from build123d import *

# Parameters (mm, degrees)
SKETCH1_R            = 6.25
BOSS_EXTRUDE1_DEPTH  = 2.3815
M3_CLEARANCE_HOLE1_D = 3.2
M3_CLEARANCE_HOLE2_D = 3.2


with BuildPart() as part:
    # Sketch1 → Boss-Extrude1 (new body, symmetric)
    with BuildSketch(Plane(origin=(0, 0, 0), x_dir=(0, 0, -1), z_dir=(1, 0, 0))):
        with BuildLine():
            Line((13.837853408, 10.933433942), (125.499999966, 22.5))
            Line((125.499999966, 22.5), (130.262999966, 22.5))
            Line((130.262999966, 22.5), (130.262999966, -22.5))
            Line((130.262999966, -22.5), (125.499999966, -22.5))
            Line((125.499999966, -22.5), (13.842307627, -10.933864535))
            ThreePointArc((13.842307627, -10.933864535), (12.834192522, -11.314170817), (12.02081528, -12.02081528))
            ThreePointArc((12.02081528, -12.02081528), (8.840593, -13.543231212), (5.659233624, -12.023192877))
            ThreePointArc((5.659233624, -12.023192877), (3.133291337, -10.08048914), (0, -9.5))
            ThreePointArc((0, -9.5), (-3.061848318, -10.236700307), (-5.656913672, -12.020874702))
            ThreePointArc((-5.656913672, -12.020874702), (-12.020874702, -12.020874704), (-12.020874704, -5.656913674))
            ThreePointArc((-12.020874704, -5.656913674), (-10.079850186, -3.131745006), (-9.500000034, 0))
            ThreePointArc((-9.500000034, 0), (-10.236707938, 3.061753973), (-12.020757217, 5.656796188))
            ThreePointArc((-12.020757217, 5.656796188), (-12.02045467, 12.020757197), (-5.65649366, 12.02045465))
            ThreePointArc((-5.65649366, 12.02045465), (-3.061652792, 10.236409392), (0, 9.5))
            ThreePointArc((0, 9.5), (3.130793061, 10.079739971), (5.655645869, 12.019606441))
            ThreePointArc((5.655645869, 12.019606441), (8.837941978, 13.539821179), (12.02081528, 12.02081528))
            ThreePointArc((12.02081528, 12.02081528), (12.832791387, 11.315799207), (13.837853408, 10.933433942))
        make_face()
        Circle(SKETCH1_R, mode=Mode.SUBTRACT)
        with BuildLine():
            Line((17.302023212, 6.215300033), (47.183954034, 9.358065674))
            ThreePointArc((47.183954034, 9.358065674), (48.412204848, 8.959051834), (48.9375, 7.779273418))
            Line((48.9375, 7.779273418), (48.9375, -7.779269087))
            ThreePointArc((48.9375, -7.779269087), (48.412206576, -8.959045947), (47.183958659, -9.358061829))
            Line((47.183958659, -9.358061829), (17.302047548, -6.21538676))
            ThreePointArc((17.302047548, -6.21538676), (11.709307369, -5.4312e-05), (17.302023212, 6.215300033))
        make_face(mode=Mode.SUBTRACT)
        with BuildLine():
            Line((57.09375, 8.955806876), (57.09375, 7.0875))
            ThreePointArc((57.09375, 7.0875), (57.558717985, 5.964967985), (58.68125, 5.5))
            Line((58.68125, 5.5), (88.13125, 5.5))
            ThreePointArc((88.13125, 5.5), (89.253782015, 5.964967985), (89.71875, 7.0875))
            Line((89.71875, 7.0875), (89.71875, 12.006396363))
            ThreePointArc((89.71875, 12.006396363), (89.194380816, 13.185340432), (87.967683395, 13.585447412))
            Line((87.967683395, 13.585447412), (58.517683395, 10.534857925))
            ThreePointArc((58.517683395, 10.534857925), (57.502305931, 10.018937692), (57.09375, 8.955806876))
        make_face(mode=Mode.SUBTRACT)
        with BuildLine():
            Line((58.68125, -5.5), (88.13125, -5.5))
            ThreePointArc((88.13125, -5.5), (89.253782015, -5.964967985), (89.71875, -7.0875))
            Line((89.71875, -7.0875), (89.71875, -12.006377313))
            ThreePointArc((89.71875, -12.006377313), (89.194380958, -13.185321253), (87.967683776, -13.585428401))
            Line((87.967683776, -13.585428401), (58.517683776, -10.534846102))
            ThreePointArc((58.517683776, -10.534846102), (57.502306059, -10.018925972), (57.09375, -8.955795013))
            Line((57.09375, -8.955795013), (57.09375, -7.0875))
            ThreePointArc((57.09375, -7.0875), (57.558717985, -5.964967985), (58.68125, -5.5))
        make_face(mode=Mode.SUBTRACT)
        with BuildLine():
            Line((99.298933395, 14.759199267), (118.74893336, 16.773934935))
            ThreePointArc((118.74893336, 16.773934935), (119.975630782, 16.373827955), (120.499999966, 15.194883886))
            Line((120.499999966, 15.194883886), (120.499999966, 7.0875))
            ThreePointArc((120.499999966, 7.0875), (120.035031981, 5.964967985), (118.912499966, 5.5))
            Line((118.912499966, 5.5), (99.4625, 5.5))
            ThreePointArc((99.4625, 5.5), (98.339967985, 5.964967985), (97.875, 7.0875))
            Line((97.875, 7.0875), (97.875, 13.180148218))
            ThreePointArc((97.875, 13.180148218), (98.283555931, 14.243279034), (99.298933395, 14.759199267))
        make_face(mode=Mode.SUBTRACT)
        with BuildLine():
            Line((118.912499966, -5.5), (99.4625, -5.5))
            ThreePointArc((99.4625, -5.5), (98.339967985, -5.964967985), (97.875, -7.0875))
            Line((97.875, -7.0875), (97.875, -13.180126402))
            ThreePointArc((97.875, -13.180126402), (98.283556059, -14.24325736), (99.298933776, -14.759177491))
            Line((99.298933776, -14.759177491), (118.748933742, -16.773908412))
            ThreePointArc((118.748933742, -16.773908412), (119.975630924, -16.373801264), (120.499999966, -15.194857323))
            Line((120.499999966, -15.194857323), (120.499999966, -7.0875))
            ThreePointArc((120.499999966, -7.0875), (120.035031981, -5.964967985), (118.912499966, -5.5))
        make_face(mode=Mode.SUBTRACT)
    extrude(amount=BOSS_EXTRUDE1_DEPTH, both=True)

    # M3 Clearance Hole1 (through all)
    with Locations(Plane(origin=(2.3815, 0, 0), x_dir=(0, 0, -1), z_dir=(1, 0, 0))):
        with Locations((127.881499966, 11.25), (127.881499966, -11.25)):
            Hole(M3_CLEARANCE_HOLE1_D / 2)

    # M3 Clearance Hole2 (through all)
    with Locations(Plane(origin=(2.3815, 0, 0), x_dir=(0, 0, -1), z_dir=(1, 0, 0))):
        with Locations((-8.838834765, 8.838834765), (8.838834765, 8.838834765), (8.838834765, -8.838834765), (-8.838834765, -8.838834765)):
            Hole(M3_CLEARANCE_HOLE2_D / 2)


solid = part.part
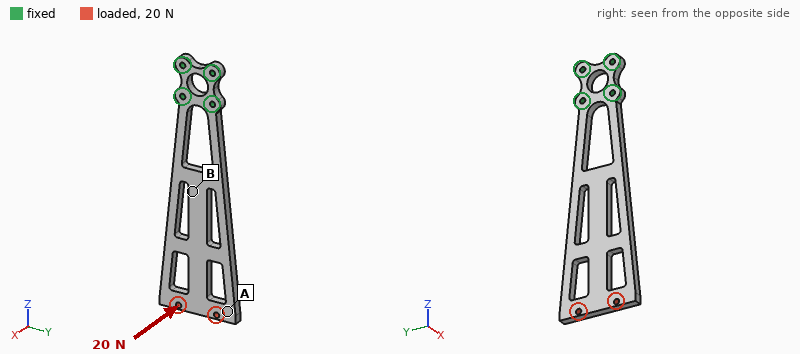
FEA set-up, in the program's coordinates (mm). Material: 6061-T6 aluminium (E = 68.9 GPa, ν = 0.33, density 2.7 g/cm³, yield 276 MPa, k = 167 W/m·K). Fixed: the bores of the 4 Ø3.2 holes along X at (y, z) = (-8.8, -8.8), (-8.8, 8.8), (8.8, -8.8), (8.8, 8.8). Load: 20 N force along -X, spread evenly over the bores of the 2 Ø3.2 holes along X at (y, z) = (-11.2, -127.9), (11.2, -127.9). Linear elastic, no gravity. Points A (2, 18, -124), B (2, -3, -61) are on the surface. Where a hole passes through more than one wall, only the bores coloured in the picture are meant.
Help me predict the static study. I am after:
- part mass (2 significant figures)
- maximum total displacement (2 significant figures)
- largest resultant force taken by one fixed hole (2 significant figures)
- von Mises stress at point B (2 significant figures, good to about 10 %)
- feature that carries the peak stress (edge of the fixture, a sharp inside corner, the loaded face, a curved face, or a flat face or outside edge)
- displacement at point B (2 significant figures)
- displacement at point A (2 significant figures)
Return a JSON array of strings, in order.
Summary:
["38 g", "1.5 mm", "15 N", "15 MPa", "a curved face", "0.40 mm", "1.4 mm"]
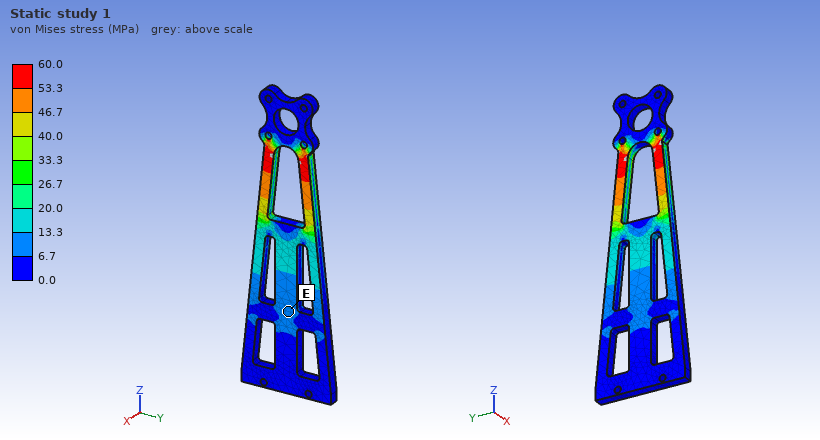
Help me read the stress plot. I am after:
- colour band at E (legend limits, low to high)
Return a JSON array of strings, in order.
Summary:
["6.7 to 13.3 MPa"]
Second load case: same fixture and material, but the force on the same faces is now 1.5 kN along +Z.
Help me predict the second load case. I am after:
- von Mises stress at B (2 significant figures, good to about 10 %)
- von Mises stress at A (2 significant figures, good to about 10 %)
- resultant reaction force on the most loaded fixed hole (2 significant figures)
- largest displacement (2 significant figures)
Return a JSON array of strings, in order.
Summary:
["13 MPa", "15 MPa", "730 N", "43 µm"]
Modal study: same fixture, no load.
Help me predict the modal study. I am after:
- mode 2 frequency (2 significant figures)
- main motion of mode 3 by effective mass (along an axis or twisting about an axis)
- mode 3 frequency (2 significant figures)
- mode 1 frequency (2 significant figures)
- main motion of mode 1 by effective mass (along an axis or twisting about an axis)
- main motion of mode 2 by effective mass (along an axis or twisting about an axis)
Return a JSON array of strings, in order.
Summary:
["610 Hz", "twisting about Z", "920 Hz", "170 Hz", "along X", "along Y"]
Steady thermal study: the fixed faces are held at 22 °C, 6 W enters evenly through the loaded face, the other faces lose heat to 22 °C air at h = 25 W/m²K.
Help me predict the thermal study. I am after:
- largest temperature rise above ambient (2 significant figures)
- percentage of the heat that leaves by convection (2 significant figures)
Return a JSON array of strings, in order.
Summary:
["30 K", "61 %"]
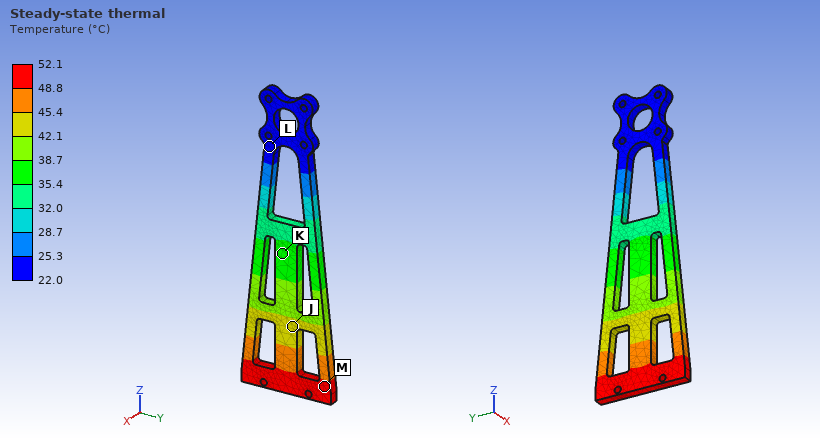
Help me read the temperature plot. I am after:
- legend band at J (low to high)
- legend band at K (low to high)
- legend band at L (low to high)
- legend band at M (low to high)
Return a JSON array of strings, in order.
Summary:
["42.1 to 45.4 °C", "35.4 to 38.7 °C", "22.0 to 25.3 °C", "48.8 to 52.1 °C"]
